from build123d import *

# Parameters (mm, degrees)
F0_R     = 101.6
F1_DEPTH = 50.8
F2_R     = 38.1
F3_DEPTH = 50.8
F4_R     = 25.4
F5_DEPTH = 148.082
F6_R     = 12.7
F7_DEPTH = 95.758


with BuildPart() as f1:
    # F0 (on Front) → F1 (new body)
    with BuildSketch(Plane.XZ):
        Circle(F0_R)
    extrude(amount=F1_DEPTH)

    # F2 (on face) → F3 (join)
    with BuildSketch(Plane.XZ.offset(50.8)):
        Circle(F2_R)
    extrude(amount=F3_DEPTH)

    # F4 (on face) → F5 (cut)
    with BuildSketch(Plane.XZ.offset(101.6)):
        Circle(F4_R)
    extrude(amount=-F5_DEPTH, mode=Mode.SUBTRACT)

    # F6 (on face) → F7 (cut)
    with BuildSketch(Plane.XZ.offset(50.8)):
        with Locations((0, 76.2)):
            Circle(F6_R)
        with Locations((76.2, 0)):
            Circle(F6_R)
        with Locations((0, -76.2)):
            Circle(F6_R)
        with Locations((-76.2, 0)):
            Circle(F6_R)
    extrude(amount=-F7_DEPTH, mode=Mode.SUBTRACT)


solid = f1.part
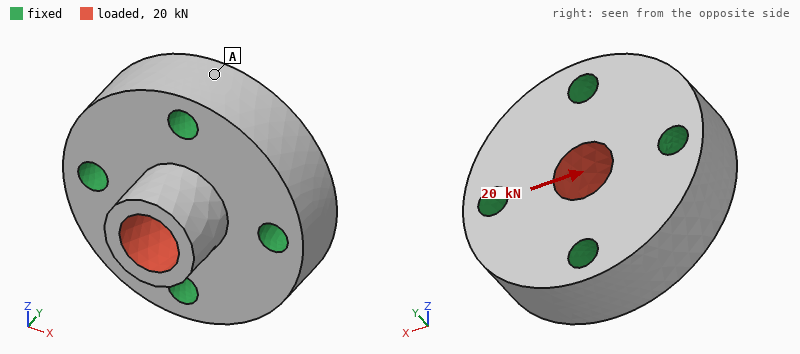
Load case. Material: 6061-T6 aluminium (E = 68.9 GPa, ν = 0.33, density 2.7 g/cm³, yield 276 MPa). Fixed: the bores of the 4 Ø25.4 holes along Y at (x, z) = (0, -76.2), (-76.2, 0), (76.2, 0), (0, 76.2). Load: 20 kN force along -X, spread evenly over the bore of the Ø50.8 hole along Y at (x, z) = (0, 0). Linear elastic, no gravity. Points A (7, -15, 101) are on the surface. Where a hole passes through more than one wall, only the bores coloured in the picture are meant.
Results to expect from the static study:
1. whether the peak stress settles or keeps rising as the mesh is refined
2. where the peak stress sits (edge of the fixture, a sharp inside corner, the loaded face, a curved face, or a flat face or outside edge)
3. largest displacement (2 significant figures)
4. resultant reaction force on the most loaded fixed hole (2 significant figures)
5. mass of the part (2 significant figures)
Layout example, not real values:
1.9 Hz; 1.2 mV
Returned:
keeps rising; a sharp inside corner; 16 µm; 7.4 kN; 4.2 kg
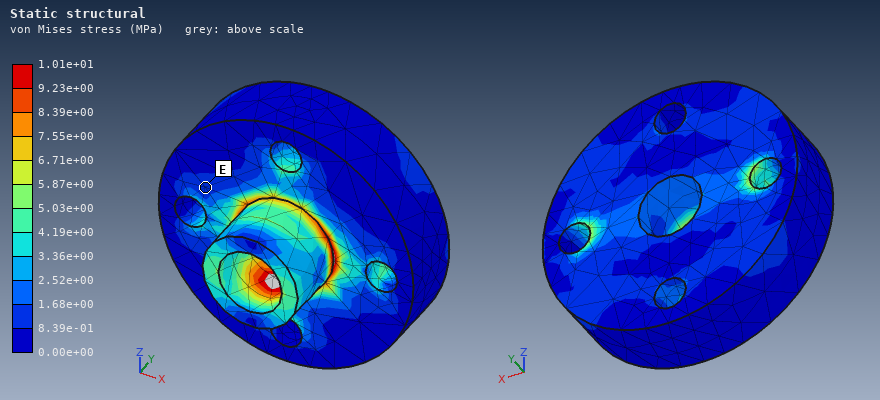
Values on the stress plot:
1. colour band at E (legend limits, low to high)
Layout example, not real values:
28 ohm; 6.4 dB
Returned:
8.39e-01 to 1.68e+00 MPa
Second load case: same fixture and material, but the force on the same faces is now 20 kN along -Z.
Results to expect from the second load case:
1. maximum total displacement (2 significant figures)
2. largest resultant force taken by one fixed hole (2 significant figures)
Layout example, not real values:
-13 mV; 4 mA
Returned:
16 µm; 7.4 kN
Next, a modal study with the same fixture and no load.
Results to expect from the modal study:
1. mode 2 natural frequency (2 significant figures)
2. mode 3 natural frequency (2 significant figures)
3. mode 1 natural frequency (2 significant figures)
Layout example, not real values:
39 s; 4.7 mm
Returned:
7900 Hz; 9800 Hz; 7900 Hz
